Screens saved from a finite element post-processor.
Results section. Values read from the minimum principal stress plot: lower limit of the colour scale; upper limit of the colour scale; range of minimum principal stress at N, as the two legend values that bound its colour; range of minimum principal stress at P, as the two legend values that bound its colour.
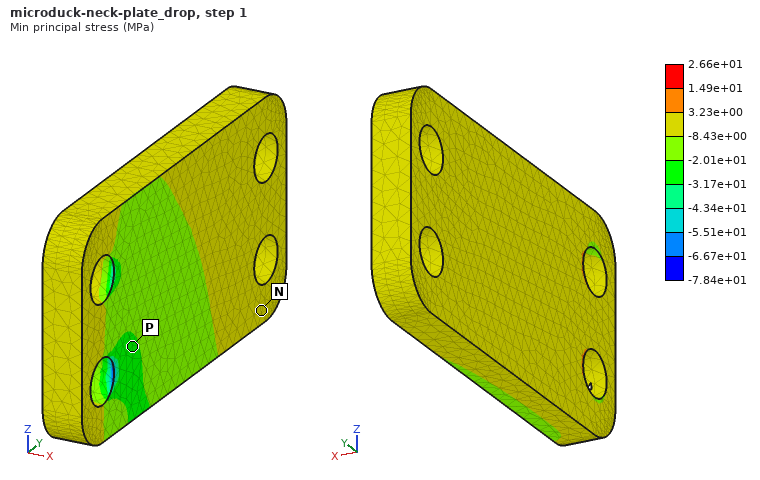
-7.84e+01 MPa
2.66e+01 MPa
-8.43e+00 to 3.23e+00 MPa
-3.17e+01 to -2.01e+01 MPa
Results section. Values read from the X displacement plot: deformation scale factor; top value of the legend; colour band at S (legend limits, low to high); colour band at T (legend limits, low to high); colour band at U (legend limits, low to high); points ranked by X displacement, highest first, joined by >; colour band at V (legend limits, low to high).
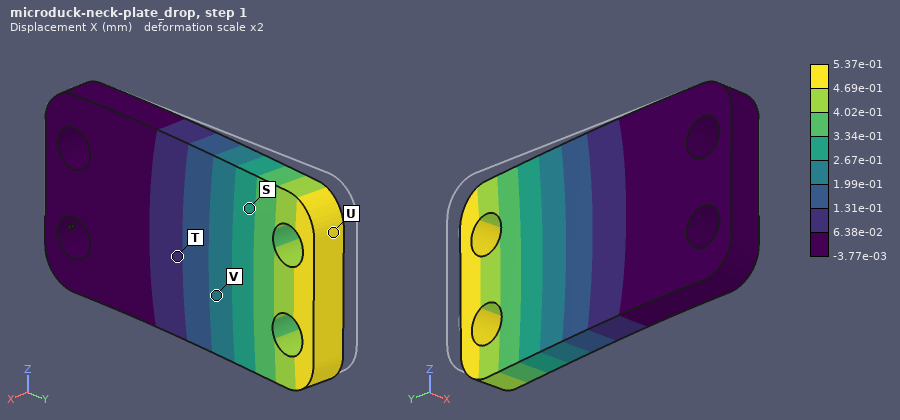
2
5.37e-01 mm
2.67e-01 to 3.34e-01 mm
6.38e-02 to 1.31e-01 mm
4.69e-01 to 5.37e-01 mm
U > S > V > T
1.99e-01 to 2.67e-01 mm
